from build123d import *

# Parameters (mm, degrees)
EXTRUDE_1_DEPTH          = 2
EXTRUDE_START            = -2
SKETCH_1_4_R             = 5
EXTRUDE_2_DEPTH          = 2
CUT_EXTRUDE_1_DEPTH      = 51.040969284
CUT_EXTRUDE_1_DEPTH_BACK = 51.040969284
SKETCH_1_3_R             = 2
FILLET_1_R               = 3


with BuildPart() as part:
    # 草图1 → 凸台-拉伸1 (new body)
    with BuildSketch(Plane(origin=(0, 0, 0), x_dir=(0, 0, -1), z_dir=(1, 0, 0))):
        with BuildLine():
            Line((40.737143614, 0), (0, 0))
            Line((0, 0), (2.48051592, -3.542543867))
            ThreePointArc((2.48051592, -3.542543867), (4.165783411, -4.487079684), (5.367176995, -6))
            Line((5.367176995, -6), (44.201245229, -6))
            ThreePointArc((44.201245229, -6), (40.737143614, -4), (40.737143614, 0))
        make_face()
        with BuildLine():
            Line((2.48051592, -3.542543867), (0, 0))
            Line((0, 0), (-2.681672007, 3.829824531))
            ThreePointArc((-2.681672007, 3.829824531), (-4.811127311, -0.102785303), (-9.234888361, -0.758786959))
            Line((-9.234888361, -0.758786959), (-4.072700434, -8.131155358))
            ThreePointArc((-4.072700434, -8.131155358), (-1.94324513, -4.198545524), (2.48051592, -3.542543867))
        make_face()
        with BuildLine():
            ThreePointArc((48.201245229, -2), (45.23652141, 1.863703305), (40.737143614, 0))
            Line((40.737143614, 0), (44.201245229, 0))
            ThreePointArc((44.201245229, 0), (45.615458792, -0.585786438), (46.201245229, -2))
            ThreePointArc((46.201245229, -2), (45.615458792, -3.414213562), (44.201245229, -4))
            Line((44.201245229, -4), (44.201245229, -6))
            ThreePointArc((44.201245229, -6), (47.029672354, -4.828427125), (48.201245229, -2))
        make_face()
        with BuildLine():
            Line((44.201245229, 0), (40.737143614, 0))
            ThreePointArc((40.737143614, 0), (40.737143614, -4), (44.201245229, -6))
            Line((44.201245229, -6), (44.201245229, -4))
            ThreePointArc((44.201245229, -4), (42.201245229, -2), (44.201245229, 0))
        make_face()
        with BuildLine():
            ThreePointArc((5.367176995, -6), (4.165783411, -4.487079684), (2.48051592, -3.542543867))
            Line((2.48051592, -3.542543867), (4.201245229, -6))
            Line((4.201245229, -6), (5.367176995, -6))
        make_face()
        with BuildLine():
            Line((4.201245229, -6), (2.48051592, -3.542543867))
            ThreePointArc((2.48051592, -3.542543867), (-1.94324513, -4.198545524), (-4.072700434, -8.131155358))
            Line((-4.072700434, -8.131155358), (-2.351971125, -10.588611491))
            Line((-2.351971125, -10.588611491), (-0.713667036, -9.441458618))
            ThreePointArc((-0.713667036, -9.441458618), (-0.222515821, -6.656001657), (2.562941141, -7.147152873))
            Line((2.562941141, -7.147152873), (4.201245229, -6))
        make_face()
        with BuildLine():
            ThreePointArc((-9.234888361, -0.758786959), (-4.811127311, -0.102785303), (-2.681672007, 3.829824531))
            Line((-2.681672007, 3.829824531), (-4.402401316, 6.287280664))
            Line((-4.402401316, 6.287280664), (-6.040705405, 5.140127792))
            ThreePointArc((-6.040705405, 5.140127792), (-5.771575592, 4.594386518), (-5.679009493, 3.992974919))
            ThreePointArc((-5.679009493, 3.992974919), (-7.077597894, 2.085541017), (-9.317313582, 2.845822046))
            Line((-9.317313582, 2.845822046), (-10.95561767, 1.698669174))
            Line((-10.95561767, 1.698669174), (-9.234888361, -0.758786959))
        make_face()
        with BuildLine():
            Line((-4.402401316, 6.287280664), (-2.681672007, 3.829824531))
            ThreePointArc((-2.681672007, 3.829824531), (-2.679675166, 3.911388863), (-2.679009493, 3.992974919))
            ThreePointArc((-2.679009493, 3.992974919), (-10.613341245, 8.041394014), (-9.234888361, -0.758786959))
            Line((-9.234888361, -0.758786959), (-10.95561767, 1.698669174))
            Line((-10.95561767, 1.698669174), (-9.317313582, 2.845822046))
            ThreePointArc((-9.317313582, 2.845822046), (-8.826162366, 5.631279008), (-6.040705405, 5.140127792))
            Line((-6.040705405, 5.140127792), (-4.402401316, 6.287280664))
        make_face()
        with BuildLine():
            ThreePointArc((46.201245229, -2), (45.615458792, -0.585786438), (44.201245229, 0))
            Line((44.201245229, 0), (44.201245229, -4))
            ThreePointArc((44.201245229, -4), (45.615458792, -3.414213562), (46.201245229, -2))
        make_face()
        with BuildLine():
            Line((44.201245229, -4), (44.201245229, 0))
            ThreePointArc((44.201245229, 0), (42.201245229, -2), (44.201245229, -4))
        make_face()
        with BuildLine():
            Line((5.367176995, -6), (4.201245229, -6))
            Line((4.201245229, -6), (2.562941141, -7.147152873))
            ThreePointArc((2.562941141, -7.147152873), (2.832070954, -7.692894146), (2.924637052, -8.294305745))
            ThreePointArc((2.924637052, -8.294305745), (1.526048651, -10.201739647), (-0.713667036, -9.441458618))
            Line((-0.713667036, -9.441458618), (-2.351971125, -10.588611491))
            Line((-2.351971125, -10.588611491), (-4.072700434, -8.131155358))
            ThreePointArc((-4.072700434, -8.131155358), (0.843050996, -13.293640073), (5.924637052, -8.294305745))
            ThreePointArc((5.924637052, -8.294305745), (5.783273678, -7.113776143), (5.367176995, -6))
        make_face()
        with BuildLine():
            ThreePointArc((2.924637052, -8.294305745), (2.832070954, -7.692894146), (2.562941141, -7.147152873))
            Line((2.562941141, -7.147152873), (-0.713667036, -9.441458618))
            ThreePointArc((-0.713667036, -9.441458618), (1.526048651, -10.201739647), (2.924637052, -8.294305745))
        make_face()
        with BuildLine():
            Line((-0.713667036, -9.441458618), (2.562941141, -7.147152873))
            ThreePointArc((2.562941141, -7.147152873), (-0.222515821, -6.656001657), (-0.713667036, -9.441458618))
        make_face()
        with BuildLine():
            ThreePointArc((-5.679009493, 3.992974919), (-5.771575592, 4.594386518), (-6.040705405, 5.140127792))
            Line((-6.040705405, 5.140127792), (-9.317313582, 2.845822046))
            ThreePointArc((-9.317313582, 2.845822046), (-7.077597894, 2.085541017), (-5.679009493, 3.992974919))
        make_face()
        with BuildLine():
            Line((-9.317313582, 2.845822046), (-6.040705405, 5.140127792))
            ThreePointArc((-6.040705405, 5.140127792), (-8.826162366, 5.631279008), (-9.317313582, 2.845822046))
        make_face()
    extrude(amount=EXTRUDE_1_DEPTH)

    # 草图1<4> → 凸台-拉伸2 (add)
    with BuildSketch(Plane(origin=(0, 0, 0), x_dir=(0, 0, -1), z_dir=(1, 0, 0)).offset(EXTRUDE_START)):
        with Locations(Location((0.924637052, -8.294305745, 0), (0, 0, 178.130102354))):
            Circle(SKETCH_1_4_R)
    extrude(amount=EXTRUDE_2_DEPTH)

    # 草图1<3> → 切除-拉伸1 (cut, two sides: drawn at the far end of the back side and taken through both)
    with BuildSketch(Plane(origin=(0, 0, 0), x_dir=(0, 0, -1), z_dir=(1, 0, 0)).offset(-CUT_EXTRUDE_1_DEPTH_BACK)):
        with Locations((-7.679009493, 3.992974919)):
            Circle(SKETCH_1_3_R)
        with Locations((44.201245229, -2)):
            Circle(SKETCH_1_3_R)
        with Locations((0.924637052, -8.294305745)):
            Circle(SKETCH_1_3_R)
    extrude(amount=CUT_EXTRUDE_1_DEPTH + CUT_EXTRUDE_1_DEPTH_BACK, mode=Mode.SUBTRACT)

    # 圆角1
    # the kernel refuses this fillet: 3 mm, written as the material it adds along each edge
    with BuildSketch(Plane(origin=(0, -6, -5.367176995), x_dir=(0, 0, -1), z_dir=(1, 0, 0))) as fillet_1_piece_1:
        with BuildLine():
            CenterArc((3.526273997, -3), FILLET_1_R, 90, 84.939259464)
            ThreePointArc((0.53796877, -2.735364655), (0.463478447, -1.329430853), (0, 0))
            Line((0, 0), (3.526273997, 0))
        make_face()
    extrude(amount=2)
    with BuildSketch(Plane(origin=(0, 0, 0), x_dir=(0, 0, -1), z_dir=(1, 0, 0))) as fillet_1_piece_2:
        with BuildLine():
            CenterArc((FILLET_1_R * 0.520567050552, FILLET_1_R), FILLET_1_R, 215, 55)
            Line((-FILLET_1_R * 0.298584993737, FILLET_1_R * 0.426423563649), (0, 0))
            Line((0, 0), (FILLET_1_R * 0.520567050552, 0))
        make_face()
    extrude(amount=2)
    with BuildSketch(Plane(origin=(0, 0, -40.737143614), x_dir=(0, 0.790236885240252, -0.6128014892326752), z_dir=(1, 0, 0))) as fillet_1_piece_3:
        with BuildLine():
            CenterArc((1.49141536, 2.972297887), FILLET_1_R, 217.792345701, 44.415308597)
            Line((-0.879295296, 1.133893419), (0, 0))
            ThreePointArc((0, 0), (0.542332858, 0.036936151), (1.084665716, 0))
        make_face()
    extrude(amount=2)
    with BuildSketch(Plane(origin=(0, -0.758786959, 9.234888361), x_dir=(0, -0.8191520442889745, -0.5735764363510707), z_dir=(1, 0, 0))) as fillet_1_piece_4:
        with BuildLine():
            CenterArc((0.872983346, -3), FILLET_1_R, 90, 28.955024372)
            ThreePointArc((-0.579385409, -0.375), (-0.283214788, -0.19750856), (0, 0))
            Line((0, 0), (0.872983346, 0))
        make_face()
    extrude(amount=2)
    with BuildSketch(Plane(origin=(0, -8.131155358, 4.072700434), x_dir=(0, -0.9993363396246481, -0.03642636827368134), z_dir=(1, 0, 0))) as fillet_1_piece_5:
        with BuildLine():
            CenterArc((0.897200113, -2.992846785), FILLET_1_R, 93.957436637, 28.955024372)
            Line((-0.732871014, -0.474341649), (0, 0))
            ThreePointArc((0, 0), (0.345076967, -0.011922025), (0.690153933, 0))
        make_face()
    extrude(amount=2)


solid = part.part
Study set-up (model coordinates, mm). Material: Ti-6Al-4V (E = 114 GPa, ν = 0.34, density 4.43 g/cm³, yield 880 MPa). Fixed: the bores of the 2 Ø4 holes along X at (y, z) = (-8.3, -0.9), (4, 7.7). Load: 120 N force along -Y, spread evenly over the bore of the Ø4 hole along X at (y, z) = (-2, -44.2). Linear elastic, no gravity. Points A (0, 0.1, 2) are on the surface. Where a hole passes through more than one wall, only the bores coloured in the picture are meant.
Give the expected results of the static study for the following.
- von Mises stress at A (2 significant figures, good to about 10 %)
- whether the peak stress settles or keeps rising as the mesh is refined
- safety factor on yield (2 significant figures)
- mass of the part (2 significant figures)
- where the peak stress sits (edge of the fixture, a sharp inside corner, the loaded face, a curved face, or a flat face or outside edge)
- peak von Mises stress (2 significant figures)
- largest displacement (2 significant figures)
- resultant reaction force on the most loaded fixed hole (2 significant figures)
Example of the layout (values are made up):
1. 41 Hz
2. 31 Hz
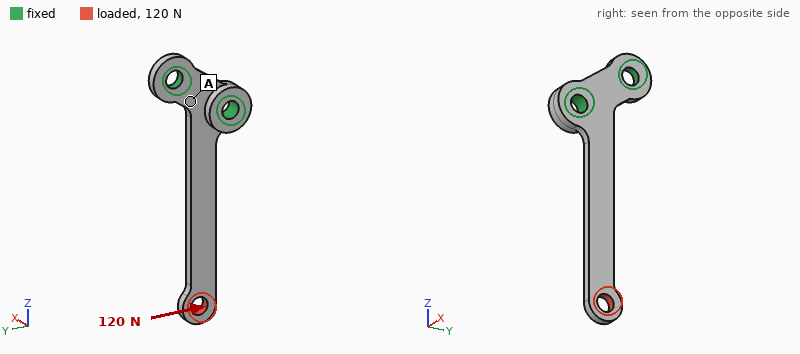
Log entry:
1. 46 MPa
2. settles
3. 1.8
4. 4.6 g
5. a curved face
6. 490 MPa
7. 0.73 mm
8. 300 N
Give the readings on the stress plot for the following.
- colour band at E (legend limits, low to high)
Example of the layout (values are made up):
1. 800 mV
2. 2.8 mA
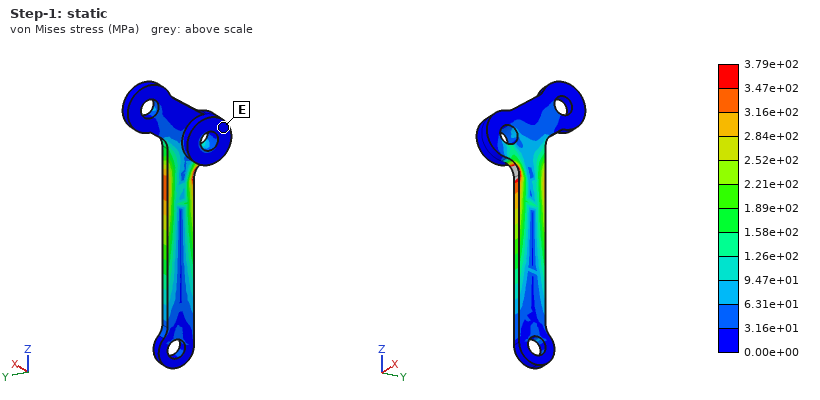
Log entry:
1. 0.00e+00 to 3.16e+01 MPa
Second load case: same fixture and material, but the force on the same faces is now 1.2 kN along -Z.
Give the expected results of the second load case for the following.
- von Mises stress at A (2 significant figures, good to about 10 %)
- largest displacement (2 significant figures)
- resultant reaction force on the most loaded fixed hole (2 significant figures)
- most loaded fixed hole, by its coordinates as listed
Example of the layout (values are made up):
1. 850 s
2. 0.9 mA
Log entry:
1. 64 MPa
2. 0.35 mm
3. 790 N
4. (-8.3, -0.9)
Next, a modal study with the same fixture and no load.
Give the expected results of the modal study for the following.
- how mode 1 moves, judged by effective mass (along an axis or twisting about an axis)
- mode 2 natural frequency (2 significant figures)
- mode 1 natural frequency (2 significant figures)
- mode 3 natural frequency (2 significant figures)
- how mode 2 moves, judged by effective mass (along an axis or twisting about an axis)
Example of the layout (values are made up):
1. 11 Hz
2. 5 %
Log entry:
1. along X
2. 2600 Hz
3. 870 Hz
4. 5300 Hz
5. along Y
